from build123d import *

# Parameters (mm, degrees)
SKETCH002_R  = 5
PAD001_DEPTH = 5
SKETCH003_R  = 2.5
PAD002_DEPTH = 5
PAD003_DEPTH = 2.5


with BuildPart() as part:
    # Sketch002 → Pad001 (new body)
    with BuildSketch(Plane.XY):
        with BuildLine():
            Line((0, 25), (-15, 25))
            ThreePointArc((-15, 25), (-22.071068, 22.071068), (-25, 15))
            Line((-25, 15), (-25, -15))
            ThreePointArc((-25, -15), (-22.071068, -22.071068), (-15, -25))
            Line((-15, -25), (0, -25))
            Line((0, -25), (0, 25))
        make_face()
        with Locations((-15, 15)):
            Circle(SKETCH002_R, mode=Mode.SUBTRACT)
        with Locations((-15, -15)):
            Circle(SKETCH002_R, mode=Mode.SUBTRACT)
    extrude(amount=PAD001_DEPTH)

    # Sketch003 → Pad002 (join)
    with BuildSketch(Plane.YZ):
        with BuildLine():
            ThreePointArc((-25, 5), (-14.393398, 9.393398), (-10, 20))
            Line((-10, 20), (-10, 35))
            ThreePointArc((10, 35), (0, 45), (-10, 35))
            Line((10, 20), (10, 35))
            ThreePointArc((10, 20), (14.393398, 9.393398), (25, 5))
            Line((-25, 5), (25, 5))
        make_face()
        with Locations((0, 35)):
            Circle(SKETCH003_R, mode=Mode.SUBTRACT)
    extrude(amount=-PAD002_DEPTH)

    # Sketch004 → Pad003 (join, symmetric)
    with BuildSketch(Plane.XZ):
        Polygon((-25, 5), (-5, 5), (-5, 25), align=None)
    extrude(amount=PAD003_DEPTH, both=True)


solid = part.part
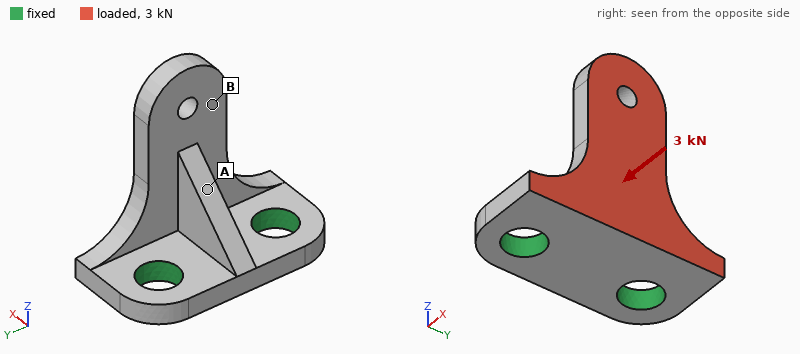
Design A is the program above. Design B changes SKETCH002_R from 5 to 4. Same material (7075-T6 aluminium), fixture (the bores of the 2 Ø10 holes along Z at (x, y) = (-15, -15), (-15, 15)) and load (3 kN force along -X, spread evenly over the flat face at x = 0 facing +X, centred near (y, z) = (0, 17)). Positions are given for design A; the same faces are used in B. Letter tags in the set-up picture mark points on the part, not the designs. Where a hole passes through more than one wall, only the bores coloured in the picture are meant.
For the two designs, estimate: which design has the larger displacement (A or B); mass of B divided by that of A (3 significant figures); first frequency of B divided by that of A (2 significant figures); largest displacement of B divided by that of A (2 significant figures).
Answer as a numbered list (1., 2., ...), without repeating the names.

1. B
2. 1.03
3. 0.93
4. 1.1
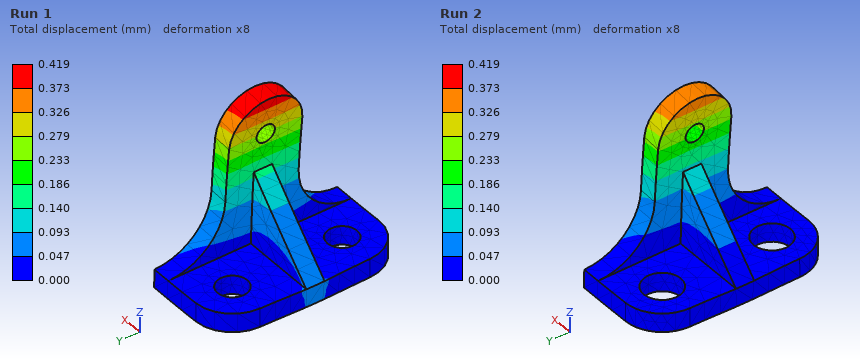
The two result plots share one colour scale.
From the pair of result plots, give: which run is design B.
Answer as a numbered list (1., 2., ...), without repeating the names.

1. Run 1
